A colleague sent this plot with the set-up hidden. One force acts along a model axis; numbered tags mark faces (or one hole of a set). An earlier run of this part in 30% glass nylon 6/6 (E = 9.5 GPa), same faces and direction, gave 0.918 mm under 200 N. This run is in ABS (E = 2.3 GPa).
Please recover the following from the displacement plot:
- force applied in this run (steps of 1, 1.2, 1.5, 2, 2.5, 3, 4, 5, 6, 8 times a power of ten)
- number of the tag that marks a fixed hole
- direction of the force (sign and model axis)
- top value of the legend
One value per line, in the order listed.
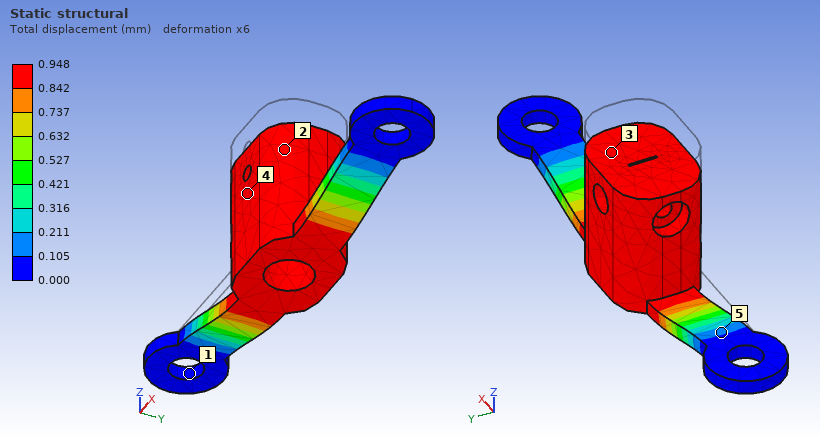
50 N
1
-Z
0.948 mm
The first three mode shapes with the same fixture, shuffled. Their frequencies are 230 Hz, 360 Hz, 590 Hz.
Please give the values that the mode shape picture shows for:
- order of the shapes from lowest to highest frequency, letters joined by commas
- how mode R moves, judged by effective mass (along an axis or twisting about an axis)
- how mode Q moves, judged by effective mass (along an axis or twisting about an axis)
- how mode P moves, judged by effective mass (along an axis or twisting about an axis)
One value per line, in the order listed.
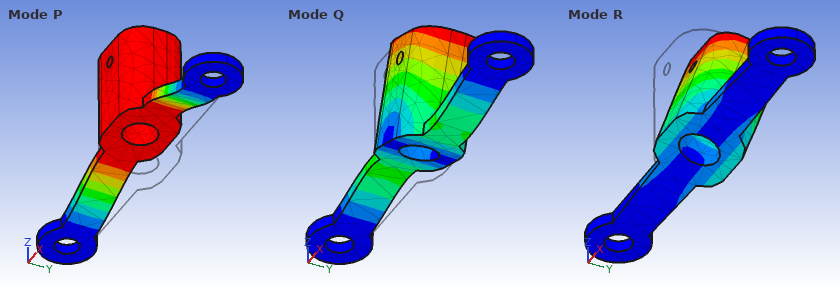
R, P, Q
along Y
along X
along Z
